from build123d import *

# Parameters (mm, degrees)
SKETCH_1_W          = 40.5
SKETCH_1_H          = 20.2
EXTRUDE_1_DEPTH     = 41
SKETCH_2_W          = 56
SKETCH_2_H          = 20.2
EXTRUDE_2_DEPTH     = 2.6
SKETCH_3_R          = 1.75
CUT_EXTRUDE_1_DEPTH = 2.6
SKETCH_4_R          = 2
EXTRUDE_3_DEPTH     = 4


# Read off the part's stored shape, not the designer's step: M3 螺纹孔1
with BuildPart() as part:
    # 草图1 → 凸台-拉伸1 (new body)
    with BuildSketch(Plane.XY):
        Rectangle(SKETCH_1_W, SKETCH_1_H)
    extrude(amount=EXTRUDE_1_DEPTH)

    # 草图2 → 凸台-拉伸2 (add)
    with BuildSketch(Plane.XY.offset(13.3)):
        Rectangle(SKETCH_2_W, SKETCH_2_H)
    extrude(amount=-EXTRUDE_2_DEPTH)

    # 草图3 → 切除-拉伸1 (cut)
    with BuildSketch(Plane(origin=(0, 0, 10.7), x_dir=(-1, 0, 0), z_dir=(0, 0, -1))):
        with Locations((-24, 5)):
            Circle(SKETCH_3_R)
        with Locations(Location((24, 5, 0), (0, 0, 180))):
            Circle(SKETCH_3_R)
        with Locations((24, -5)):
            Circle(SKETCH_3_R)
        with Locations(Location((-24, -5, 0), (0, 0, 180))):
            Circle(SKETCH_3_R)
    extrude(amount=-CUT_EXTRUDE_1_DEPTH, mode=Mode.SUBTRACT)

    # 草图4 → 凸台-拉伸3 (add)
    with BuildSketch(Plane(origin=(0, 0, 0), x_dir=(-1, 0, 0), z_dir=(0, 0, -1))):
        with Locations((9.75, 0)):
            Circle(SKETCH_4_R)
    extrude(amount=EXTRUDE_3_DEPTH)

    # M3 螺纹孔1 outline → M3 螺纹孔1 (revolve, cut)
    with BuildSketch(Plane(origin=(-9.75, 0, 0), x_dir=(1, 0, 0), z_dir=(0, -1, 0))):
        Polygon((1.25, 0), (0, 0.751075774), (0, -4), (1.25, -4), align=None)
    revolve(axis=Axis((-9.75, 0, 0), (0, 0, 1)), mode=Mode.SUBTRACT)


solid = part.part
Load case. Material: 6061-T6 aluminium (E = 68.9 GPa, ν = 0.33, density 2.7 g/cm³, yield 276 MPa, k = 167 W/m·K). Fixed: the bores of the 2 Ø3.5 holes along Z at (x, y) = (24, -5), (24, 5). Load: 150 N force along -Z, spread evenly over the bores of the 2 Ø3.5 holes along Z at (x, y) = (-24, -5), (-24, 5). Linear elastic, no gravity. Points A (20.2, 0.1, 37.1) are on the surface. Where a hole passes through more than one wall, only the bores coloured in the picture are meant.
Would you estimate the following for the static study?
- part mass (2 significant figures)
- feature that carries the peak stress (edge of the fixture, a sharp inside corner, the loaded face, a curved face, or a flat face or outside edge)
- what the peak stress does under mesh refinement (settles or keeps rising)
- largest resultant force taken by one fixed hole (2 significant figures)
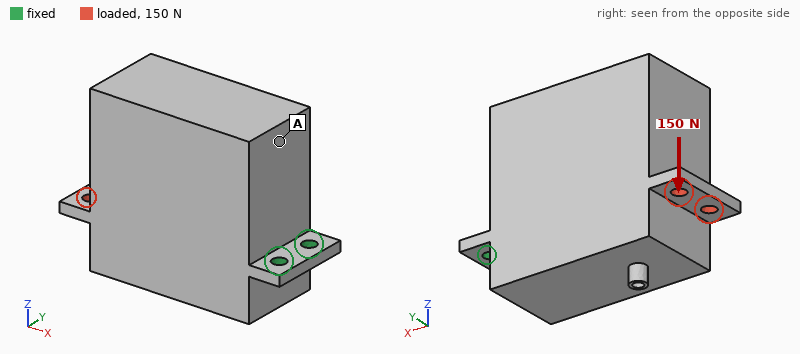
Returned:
93 g
edge of the fixture
keeps rising
76 N
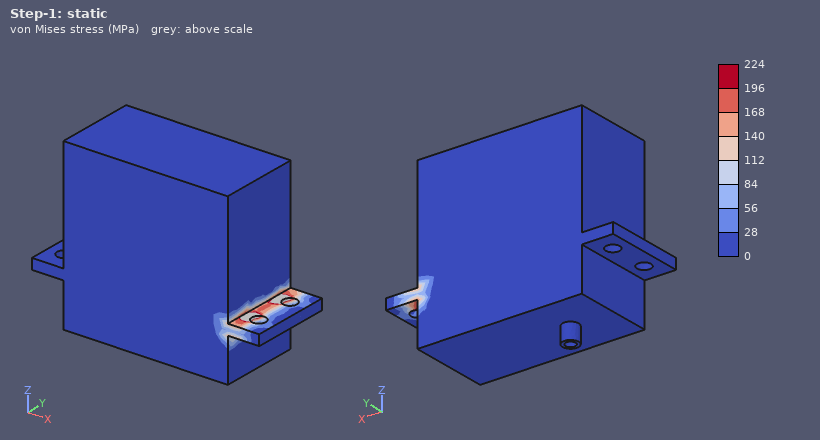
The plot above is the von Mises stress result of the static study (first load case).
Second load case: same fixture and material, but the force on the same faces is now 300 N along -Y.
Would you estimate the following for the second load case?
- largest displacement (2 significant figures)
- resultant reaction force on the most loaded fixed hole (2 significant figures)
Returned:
54 µm
1.2 kN
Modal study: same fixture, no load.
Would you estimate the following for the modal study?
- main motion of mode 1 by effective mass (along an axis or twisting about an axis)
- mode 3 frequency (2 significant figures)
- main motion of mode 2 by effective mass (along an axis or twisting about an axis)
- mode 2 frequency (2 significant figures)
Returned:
along Z
3300 Hz
along Y
2000 Hz
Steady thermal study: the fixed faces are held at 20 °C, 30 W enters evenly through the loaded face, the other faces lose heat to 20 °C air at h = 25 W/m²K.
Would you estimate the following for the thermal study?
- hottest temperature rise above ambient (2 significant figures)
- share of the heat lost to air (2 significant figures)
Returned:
51 K
12 %
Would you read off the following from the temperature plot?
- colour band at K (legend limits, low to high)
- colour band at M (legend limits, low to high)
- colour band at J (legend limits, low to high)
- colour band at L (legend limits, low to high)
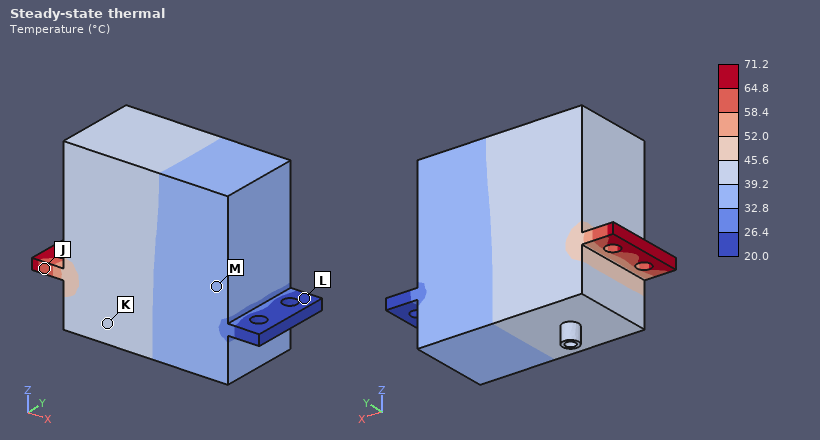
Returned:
39.2 to 45.6 °C
32.8 to 39.2 °C
58.4 to 64.8 °C
20.0 to 26.4 °C
